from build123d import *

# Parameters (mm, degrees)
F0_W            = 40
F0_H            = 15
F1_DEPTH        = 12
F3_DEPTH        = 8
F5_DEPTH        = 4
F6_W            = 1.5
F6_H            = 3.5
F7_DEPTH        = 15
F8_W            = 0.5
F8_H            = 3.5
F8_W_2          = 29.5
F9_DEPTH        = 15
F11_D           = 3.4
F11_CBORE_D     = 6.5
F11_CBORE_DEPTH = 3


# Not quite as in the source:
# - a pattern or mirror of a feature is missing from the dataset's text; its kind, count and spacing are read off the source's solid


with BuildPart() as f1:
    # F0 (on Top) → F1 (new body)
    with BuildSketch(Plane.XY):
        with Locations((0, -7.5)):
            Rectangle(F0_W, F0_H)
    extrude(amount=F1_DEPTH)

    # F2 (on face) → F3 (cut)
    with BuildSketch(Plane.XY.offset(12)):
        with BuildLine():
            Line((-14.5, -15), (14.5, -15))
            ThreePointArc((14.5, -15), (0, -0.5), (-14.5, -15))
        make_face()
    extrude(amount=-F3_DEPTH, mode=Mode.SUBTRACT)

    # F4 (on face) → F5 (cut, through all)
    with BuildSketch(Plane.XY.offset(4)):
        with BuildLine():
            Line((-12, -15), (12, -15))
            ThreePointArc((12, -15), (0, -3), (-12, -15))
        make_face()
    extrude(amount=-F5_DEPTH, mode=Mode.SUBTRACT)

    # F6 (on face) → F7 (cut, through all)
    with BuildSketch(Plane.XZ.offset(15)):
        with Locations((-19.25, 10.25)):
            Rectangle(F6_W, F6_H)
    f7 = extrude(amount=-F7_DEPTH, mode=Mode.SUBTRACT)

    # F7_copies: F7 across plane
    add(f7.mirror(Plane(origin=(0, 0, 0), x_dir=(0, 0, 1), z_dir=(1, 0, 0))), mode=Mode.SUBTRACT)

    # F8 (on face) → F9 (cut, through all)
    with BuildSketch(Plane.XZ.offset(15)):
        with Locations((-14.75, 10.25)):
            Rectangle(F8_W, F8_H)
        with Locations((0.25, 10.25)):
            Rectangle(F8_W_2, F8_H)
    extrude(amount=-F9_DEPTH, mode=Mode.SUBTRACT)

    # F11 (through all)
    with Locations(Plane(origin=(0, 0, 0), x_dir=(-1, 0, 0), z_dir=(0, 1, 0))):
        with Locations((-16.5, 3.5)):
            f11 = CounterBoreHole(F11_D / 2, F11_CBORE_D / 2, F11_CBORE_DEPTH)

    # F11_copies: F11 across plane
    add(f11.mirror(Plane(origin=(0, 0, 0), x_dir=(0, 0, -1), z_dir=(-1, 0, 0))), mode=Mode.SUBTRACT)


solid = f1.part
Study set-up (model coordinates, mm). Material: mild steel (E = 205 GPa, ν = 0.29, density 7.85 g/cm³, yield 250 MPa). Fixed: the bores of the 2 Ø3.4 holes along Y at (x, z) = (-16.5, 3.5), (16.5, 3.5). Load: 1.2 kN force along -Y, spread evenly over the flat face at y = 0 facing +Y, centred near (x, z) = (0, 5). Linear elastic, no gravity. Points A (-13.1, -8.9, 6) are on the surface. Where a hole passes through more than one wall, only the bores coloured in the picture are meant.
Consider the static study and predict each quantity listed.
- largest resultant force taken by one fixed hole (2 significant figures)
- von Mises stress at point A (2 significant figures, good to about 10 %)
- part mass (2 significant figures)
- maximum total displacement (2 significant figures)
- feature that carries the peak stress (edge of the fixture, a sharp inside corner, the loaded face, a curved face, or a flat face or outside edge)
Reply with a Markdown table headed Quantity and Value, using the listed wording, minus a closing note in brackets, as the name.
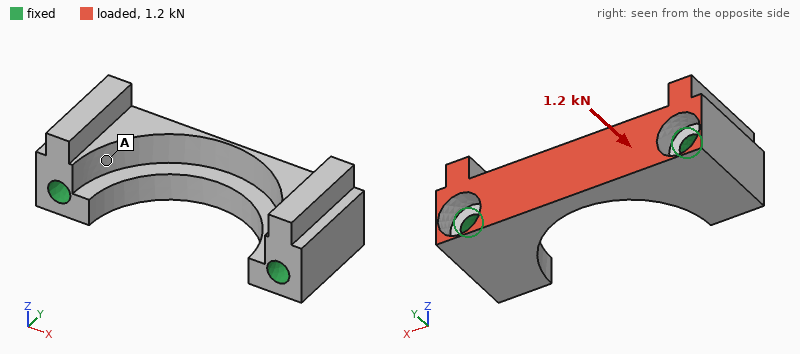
| Quantity | Value |
|---|---|
| largest resultant force taken by one fixed hole | 700 N |
| von Mises stress at point A | 17 MPa |
| part mass | 21 g |
| maximum total displacement | 14 µm |
| feature that carries the peak stress | the loaded face |
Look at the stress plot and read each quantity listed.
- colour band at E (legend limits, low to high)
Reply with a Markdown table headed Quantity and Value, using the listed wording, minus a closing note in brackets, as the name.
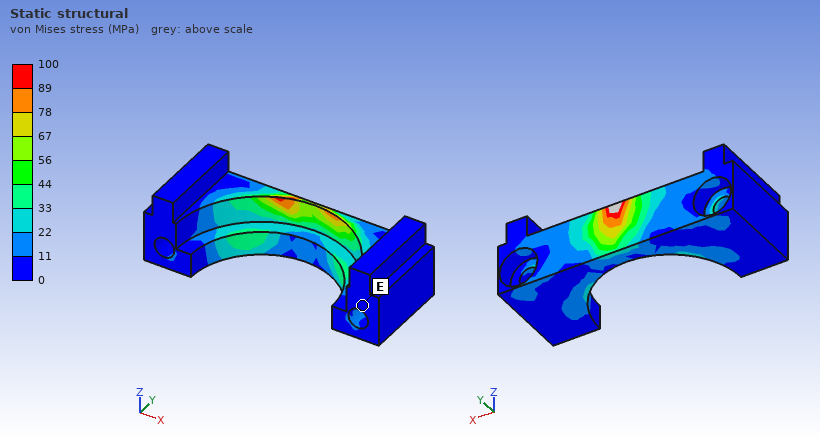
| Quantity | Value |
|---|---|
| colour band at E | 0 to 11 MPa |
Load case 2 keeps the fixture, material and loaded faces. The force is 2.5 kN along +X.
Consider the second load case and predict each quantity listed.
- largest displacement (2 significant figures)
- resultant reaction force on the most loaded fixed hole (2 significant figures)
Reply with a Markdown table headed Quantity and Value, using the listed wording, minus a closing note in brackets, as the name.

| Quantity | Value |
|---|---|
| largest displacement | 6.3 µm |
| resultant reaction force on the most loaded fixed hole | 1.3 kN |
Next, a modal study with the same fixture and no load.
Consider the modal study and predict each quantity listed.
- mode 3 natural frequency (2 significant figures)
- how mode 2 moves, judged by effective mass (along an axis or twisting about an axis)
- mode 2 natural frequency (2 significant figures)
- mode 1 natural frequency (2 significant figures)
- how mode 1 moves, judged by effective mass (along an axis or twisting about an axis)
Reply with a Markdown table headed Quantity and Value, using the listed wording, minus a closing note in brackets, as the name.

| Quantity | Value |
|---|---|
| mode 3 natural frequency | 47 kHz |
| how mode 2 moves, judged by effective mass | along Y |
| mode 2 natural frequency | 43 kHz |
| mode 1 natural frequency | 31 kHz |
| how mode 1 moves, judged by effective mass | along Z |
